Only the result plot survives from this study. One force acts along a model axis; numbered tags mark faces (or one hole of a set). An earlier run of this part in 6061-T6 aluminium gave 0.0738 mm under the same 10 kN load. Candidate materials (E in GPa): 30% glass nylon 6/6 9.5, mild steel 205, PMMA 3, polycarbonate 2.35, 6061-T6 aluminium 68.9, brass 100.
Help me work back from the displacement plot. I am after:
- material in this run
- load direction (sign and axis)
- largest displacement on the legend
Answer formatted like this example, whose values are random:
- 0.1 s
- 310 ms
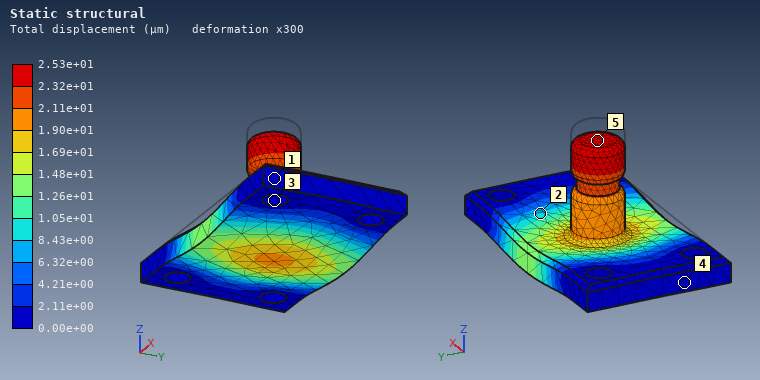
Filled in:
- mild steel
- -Z
- 2.53e+01 µm
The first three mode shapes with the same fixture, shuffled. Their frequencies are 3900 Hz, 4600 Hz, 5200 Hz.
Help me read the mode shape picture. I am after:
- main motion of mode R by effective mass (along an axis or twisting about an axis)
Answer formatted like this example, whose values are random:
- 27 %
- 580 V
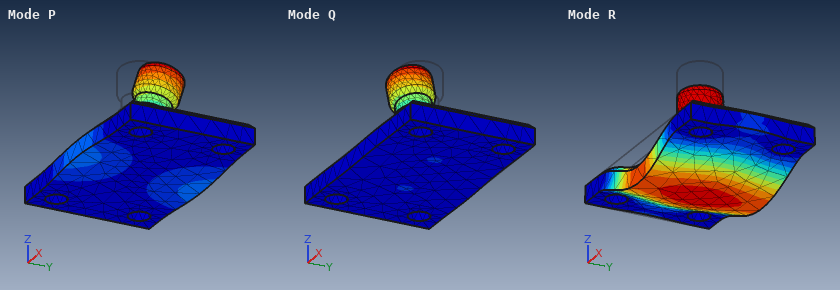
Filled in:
- along Z
